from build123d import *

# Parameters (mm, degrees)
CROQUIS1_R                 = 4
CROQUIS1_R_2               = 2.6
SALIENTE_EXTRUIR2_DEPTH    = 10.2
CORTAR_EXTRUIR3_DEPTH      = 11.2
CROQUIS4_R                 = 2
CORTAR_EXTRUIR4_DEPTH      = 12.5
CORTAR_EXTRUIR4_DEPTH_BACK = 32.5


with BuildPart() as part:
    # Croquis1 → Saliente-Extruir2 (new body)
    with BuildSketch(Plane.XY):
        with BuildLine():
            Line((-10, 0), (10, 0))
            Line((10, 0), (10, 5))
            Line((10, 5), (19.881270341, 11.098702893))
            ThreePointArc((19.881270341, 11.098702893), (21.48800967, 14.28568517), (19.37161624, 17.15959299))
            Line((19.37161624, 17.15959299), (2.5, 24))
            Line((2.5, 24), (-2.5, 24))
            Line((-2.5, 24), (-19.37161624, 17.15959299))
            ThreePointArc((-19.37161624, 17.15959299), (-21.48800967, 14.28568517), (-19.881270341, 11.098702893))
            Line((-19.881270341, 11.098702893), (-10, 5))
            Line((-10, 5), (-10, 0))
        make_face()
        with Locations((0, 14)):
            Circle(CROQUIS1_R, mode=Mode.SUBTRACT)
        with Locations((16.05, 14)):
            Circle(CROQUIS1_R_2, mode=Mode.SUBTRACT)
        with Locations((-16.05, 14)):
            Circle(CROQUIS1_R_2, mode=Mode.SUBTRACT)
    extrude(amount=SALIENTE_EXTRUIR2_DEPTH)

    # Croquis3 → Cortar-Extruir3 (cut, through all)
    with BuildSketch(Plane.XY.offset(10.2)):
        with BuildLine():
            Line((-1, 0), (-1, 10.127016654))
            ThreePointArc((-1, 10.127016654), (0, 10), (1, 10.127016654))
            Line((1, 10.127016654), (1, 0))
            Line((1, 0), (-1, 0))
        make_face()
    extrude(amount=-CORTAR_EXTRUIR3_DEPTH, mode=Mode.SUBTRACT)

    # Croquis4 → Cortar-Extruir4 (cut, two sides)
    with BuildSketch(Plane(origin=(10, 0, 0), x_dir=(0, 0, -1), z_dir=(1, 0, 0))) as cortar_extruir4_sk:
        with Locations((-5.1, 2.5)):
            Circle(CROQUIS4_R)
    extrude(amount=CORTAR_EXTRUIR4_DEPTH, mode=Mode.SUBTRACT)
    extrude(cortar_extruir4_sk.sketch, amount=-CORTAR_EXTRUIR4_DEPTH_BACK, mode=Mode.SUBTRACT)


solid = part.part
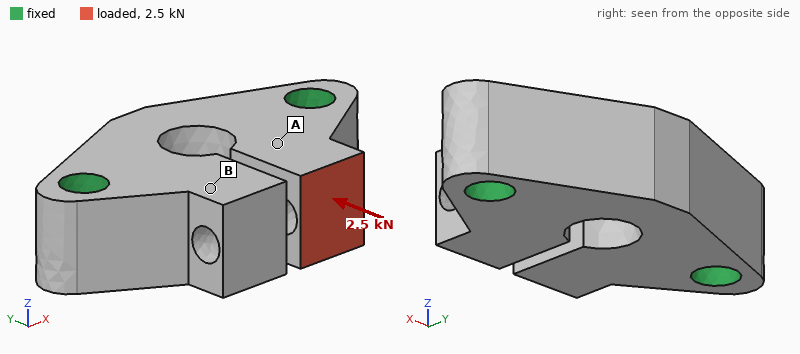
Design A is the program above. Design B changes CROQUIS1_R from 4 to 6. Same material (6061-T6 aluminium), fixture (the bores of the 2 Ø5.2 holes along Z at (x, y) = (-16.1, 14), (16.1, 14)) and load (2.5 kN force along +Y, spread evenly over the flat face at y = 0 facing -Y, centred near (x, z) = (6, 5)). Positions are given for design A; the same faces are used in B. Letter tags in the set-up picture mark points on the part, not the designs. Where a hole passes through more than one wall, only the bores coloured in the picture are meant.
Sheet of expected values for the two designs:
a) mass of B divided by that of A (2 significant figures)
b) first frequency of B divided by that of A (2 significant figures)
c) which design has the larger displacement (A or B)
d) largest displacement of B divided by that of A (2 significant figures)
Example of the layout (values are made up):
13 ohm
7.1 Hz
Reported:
0.89
0.95
B
1.5
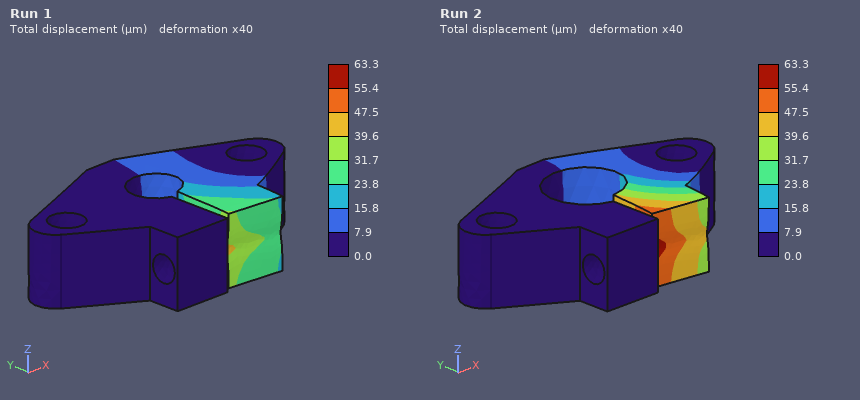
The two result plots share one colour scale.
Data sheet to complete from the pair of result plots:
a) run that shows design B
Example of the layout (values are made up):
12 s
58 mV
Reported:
Run 2
